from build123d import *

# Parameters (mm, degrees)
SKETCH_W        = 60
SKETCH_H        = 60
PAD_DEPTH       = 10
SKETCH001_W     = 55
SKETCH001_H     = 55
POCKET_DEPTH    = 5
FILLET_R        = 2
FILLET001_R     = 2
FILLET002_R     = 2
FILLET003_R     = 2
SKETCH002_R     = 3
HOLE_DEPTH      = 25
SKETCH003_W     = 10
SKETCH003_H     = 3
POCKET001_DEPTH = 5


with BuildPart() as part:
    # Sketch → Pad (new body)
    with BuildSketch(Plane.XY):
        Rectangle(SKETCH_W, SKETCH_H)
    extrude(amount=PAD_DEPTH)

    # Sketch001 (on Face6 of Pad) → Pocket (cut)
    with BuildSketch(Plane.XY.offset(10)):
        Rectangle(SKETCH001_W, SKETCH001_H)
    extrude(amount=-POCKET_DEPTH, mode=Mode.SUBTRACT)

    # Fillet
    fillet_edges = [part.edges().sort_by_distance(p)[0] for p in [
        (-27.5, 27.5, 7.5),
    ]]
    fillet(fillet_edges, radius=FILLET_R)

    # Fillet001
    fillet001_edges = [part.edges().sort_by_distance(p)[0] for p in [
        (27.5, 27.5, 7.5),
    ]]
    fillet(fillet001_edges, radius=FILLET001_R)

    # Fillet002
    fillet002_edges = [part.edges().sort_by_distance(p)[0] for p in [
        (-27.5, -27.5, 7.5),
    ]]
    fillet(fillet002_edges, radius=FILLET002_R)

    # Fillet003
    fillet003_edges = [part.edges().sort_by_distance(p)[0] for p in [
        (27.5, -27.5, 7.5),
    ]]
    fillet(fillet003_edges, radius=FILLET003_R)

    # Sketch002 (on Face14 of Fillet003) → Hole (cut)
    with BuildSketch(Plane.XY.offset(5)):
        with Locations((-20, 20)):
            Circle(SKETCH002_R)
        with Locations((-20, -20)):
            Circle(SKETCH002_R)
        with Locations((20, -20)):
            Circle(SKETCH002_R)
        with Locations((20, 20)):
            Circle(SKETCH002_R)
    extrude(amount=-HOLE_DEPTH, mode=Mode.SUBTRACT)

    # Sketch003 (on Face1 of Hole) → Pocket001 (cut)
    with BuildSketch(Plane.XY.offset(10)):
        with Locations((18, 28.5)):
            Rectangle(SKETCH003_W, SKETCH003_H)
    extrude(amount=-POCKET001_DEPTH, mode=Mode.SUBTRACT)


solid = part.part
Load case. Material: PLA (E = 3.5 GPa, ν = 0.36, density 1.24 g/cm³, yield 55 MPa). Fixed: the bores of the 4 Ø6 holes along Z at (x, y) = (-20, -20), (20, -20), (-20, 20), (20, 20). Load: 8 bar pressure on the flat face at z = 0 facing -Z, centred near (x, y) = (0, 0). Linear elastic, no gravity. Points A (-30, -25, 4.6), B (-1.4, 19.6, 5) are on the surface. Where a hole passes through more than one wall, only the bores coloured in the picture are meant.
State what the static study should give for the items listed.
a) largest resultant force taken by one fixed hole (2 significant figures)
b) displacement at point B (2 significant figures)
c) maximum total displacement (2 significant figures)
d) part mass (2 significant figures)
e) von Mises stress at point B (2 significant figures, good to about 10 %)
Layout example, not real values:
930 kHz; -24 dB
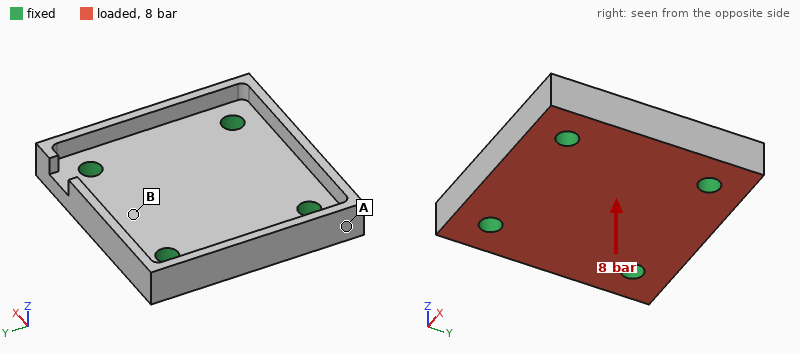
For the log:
700 N; 0.15 mm; 0.27 mm; 25 g; 9.9 MPa
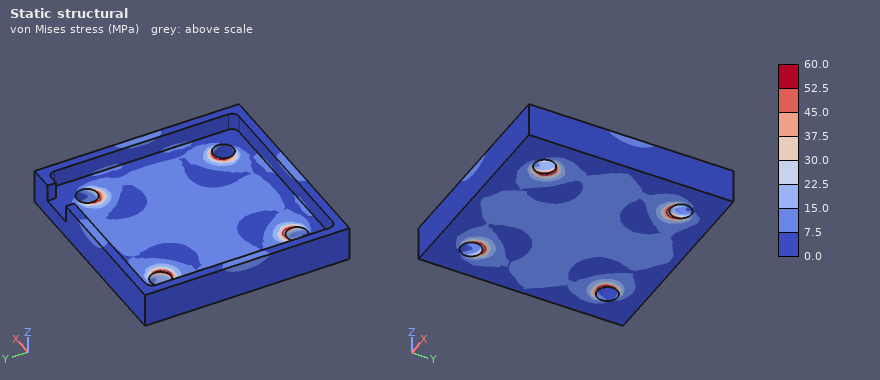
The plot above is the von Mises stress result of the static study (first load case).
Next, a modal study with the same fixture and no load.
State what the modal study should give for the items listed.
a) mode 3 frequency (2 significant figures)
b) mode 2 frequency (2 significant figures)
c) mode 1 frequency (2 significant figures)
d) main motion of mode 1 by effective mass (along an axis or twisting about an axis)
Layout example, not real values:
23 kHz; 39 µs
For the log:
5700 Hz; 5600 Hz; 4200 Hz; along Z
